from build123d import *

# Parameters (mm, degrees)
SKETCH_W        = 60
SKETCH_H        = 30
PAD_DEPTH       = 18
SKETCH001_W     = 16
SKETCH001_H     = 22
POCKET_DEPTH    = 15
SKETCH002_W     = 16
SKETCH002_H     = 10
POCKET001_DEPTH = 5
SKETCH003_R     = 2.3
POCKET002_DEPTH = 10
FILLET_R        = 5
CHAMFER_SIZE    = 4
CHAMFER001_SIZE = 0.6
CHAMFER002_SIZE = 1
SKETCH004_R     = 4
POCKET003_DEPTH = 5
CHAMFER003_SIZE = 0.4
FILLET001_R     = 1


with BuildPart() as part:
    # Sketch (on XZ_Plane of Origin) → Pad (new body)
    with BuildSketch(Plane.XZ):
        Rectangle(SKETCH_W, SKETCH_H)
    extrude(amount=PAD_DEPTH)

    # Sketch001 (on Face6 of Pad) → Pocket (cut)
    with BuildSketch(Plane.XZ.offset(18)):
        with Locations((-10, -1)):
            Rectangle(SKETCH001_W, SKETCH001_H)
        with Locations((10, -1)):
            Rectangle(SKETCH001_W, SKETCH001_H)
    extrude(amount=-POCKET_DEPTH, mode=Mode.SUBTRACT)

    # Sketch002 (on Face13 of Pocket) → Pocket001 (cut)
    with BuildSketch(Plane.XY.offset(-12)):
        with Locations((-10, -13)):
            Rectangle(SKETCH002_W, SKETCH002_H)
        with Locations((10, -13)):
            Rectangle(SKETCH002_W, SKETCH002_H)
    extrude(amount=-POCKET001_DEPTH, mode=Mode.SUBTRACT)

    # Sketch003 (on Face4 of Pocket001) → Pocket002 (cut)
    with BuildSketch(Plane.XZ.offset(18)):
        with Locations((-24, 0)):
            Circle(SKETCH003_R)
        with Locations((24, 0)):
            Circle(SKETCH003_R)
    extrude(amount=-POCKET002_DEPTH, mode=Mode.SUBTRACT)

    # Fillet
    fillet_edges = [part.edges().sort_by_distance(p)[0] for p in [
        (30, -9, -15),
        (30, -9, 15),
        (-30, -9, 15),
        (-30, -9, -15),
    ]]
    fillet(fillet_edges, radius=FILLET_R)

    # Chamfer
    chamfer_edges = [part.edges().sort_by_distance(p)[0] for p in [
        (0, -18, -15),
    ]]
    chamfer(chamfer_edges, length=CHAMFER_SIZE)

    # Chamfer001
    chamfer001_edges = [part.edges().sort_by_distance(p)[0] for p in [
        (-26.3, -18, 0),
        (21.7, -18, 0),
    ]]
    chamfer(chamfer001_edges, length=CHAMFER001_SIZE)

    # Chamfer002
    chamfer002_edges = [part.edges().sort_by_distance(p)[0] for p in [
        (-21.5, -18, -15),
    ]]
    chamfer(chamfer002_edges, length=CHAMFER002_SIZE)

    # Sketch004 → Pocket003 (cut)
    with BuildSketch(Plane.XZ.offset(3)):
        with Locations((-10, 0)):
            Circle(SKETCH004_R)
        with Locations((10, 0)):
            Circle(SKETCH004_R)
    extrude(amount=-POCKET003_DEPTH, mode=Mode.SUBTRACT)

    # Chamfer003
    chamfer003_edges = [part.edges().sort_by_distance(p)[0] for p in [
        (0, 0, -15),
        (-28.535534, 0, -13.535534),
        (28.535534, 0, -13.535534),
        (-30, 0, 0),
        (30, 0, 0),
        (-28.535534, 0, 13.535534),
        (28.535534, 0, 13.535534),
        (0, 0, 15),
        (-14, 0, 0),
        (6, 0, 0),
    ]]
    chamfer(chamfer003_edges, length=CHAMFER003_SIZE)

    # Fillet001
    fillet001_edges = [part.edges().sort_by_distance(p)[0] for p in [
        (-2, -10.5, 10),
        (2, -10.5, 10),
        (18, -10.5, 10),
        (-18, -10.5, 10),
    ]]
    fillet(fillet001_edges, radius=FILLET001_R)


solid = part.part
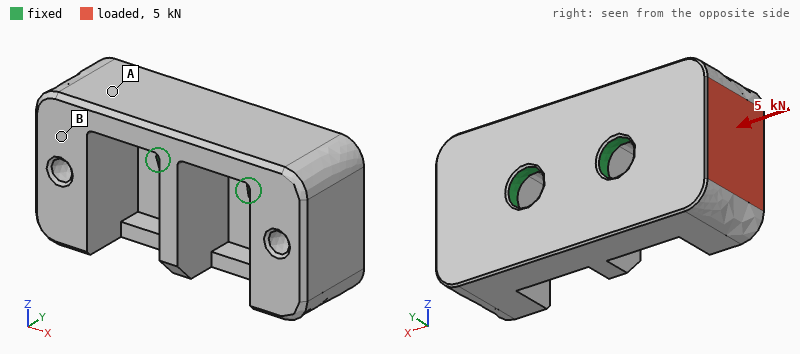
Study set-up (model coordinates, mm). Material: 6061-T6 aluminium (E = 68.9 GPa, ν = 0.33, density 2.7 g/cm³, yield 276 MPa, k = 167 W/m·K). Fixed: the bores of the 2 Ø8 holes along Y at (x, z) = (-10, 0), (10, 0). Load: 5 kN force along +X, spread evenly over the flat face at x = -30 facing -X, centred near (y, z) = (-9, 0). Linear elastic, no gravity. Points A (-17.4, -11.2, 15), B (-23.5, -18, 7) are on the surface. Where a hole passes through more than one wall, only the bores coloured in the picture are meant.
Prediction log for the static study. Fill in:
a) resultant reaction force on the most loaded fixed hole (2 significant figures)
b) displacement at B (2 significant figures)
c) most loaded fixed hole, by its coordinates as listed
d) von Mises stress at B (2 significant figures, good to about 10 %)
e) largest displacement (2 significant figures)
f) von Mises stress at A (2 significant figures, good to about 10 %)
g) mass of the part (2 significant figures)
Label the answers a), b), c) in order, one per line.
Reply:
a) 3.3 kN
b) 0.090 mm
c) (-10, 0)
d) 56 MPa
e) 0.12 mm
f) 21 MPa
g) 53 g
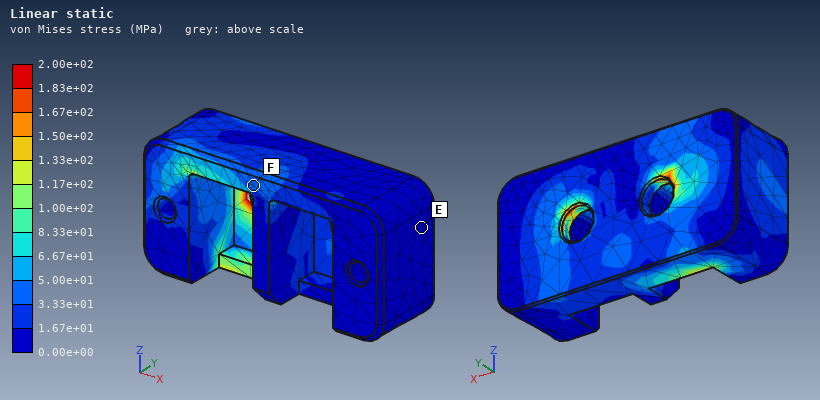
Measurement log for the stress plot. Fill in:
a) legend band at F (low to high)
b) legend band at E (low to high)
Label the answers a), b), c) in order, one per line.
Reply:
a) 3.33e+01 to 5.00e+01 MPa
b) 0.00e+00 to 1.67e+01 MPa
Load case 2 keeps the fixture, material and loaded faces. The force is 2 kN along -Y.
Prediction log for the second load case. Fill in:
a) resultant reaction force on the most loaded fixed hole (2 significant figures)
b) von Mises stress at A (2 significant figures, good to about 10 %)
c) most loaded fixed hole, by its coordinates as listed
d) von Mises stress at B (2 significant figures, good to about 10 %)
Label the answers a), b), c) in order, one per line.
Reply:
a) 3.3 kN
b) 19 MPa
c) (-10, 0)
d) 43 MPa
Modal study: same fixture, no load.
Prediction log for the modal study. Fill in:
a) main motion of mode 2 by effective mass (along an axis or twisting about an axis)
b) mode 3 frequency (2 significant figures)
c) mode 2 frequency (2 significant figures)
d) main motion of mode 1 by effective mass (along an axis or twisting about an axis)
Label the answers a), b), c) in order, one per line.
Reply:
a) along X
b) 7400 Hz
c) 5200 Hz
d) along Z
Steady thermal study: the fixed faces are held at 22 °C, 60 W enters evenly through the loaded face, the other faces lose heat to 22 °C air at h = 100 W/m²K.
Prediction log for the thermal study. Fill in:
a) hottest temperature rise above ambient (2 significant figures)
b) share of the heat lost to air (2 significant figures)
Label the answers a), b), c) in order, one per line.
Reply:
a) 38 K
b) 15 %
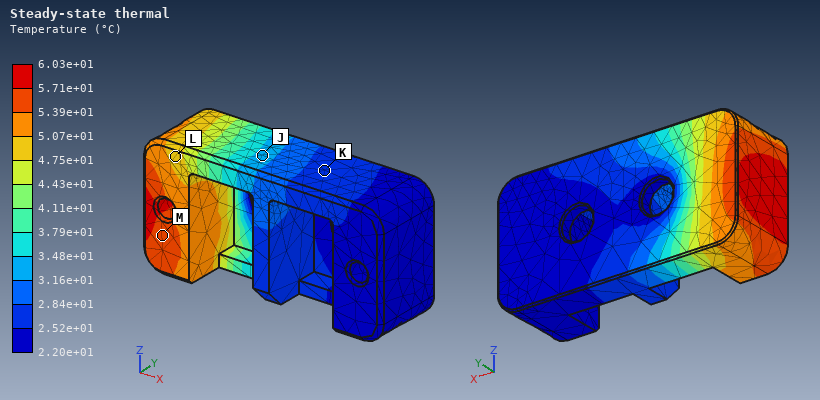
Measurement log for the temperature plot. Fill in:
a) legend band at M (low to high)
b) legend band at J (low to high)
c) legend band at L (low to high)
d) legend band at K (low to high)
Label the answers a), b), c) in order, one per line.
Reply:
a) 5.39e+01 to 5.71e+01 °C
b) 3.16e+01 to 3.48e+01 °C
c) 4.75e+01 to 5.07e+01 °C
d) 2.52e+01 to 2.84e+01 °C
